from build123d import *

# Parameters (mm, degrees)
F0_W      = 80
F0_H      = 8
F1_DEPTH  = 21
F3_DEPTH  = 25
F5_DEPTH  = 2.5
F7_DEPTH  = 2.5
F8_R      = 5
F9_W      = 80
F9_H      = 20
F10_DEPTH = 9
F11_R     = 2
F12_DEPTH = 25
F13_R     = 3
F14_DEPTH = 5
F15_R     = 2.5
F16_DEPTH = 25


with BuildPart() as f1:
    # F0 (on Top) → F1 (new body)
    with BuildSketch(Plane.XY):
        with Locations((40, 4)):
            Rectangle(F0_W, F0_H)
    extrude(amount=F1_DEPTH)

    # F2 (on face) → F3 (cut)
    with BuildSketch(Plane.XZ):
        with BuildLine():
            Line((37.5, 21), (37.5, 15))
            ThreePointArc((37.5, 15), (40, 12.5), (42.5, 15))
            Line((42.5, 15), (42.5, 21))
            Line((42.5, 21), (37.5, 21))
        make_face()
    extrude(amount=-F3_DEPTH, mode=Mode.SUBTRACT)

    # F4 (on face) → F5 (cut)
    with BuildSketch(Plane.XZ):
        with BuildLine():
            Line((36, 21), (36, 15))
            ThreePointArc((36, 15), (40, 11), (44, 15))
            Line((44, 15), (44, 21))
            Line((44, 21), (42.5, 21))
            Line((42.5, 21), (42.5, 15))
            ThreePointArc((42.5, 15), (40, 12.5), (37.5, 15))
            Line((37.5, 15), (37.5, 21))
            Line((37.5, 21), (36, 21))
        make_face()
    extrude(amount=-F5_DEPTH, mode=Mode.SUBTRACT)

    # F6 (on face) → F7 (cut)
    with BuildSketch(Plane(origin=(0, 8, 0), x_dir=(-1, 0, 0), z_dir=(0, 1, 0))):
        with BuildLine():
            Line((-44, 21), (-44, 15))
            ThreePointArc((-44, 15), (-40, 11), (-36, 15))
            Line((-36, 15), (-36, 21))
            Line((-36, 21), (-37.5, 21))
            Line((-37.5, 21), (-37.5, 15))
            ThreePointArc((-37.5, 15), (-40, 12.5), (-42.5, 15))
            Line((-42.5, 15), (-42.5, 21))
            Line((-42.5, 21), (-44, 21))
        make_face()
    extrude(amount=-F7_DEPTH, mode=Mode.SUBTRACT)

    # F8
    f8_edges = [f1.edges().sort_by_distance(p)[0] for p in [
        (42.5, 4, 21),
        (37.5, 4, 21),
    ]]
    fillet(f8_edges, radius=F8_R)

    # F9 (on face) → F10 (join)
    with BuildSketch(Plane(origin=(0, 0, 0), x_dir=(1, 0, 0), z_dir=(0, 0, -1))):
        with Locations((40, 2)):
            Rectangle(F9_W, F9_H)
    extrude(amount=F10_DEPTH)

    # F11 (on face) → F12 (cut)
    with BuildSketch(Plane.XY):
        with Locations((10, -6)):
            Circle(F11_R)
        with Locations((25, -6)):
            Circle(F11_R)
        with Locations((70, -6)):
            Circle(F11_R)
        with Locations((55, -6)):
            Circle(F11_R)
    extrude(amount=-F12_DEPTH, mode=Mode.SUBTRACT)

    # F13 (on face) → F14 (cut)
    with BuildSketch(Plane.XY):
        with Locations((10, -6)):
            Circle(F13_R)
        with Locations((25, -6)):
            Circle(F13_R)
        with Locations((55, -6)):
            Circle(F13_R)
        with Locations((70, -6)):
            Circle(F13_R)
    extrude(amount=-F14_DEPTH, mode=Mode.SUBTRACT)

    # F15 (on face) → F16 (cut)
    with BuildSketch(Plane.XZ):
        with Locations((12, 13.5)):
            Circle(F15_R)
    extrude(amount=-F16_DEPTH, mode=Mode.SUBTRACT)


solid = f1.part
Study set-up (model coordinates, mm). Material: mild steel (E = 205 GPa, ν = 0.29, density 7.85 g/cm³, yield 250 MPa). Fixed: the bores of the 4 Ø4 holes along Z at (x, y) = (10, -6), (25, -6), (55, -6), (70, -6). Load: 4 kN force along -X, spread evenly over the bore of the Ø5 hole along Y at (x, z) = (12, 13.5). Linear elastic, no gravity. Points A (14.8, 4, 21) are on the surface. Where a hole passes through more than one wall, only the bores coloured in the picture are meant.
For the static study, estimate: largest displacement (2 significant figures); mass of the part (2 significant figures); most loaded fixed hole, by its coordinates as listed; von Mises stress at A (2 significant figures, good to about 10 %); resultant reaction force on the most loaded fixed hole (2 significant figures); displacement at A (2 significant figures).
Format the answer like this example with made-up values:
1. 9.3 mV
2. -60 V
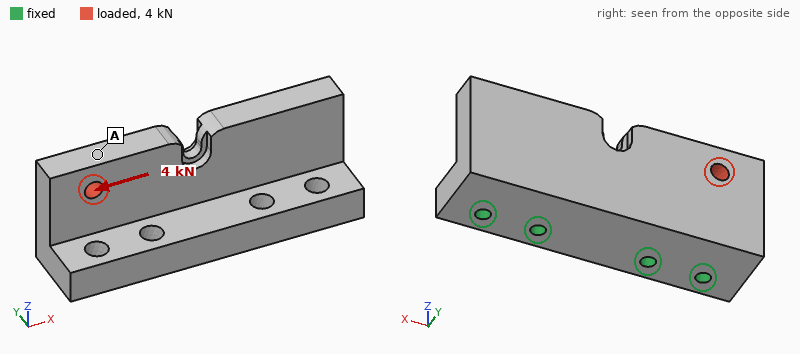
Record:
1. 16 µm
2. 210 g
3. (10, -6)
4. 16 MPa
5. 2.0 kN
6. 12 µm
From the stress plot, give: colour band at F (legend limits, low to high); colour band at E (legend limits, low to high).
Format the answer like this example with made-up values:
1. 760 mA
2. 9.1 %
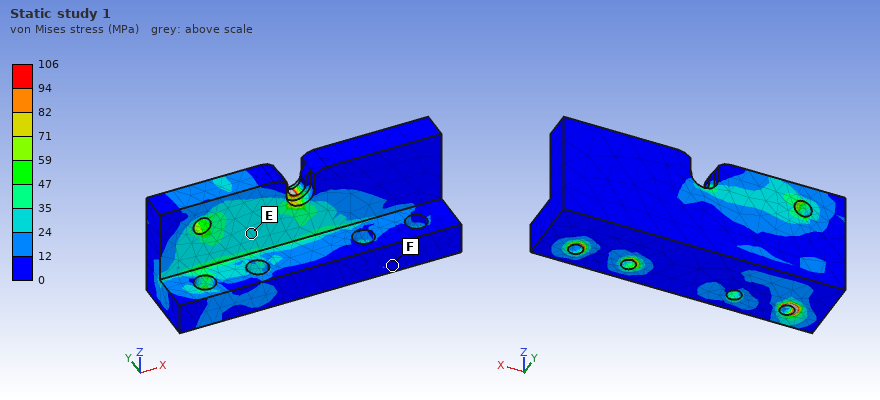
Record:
1. 0 to 12 MPa
2. 24 to 35 MPa
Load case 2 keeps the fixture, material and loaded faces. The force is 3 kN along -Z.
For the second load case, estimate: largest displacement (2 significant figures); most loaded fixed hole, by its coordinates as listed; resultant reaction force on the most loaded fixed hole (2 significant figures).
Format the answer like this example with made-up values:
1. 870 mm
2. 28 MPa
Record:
1. 37 µm
2. (10, -6)
3. 2.1 kN
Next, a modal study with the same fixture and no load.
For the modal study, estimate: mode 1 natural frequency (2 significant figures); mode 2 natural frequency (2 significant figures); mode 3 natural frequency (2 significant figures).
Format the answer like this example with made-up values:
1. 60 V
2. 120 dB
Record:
1. 4300 Hz
2. 6700 Hz
3. 13 kHz
